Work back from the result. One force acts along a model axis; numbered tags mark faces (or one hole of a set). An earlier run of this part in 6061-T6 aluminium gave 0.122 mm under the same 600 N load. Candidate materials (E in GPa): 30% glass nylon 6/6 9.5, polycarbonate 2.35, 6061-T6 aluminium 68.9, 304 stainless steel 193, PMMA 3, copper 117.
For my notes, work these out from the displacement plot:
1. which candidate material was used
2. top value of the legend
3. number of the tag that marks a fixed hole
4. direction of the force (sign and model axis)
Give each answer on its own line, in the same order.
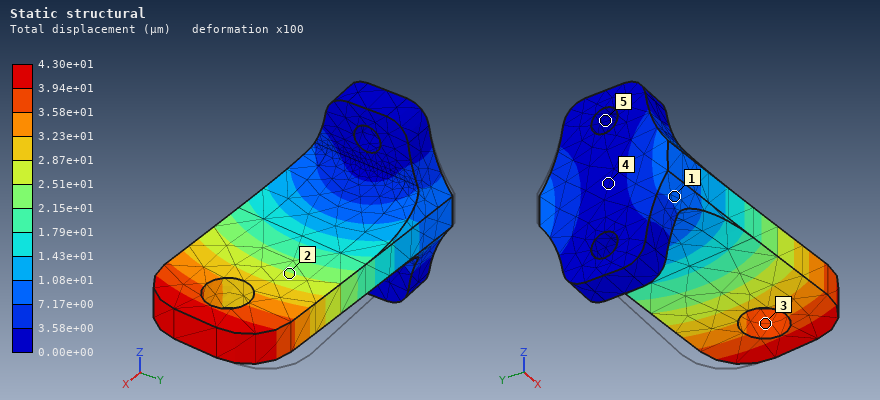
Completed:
304 stainless steel
4.30e+01 µm
5
-Y
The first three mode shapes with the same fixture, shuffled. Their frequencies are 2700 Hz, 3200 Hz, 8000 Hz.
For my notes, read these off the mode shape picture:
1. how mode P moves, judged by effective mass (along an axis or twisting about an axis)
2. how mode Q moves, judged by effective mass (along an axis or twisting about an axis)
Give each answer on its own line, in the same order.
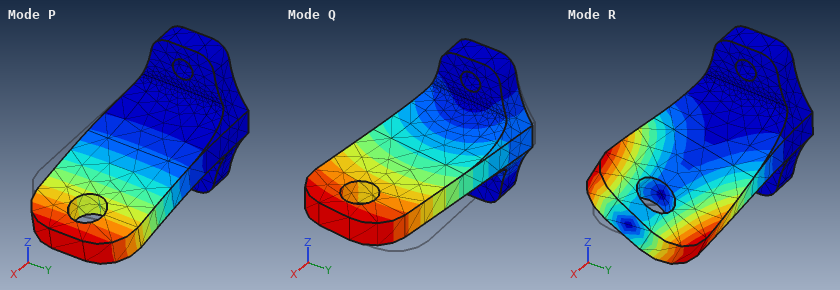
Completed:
along Z
along Y
